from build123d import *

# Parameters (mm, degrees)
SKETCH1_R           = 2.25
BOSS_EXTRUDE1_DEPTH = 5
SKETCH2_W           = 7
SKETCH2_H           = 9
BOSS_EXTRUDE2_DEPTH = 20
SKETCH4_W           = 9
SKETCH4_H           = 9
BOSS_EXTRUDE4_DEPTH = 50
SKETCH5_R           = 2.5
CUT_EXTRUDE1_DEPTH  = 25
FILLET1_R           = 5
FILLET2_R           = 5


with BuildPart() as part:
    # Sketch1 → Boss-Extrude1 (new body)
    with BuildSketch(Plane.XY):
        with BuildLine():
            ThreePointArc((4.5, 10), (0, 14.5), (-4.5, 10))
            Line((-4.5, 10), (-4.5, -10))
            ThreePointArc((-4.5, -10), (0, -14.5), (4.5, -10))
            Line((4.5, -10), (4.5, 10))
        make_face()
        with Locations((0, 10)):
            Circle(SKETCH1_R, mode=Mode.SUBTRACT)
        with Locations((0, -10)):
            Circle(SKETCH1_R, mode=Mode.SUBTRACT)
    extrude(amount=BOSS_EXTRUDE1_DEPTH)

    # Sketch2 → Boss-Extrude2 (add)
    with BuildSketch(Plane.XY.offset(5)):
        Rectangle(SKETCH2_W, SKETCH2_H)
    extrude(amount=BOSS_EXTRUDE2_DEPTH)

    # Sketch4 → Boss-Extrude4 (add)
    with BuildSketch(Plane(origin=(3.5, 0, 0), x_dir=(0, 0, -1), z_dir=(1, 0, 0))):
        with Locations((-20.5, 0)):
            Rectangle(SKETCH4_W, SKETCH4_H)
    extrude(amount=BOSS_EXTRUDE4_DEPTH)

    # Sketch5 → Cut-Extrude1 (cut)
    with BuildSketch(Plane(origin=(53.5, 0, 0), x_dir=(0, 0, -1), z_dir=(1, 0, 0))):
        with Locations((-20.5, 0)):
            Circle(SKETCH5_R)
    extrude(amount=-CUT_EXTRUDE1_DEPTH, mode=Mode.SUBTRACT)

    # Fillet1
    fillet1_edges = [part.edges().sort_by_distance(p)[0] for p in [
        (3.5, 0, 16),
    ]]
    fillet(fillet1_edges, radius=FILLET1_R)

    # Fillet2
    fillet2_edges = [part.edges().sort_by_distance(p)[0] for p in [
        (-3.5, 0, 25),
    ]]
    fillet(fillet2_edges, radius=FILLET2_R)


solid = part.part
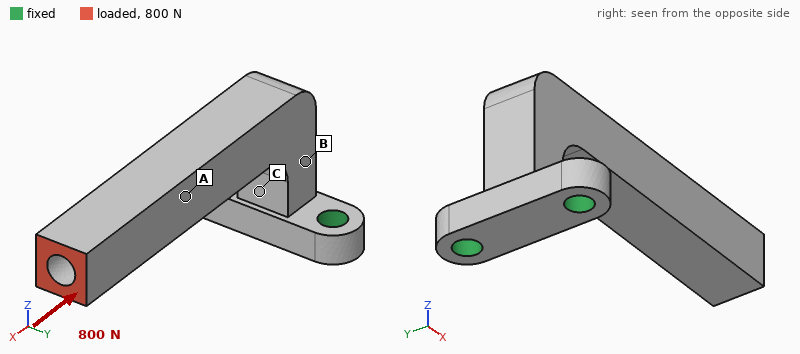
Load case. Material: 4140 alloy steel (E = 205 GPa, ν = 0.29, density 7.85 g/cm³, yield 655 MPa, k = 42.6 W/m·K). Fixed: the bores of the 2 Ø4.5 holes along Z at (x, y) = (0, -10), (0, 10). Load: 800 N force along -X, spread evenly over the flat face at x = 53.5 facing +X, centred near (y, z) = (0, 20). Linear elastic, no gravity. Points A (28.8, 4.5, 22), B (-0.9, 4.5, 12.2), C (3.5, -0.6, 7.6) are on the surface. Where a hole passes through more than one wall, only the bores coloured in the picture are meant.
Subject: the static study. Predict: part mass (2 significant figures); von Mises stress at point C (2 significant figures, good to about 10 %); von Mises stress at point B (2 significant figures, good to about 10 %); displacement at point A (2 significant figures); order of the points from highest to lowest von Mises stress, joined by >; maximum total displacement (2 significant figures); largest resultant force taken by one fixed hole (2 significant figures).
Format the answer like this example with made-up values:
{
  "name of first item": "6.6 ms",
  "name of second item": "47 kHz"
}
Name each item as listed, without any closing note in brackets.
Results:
{
  "part mass": "46 g",
  "von Mises stress at point C": "130 MPa",
  "von Mises stress at point B": "50 MPa",
  "displacement at point A": "0.12 mm",
  "order of the points from highest to lowest von Mises stress, joined by >": "C > B > A",
  "maximum total displacement": "0.21 mm",
  "largest resultant force taken by one fixed hole": "400 N"
}
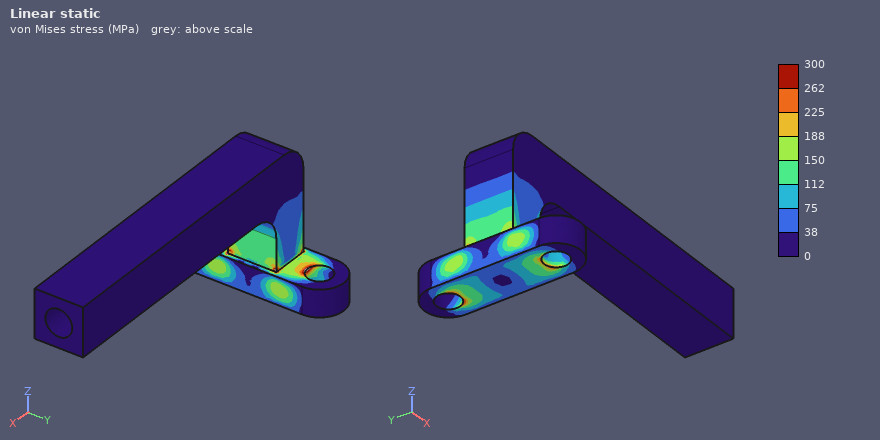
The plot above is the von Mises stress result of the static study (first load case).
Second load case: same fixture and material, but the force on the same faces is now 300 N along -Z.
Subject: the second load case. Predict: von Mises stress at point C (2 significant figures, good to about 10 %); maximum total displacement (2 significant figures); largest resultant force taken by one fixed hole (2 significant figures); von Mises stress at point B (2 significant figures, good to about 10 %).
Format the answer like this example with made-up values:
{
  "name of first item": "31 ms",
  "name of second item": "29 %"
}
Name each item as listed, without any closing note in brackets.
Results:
{
  "von Mises stress at point C": "200 MPa",
  "maximum total displacement": "0.44 mm",
  "largest resultant force taken by one fixed hole": "150 N",
  "von Mises stress at point B": "68 MPa"
}
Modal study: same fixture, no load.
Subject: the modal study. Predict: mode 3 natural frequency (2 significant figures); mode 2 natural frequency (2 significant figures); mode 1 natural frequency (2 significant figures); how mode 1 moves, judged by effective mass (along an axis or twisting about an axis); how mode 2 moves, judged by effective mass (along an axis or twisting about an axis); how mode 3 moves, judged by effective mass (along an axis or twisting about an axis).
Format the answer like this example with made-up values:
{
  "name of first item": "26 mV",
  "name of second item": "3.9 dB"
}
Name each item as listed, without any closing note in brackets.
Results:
{
  "mode 3 natural frequency": "5800 Hz",
  "mode 2 natural frequency": "1600 Hz",
  "mode 1 natural frequency": "1400 Hz",
  "how mode 1 moves, judged by effective mass": "along Z",
  "how mode 2 moves, judged by effective mass": "along Y",
  "how mode 3 moves, judged by effective mass": "along X"
}
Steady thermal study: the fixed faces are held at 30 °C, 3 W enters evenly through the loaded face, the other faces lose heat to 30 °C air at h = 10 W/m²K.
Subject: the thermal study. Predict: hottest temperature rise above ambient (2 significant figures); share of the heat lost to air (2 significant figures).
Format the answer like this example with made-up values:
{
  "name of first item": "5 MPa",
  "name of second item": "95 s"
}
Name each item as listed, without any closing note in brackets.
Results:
{
  "hottest temperature rise above ambient": "57 K",
  "share of the heat lost to air": "28 %"
}
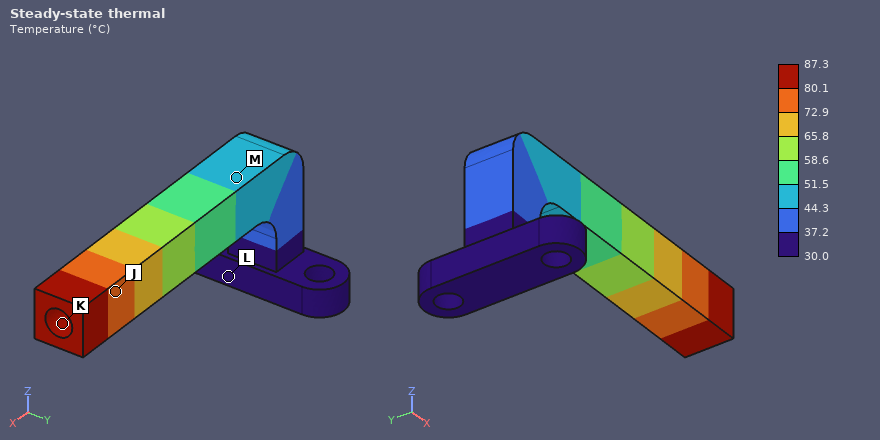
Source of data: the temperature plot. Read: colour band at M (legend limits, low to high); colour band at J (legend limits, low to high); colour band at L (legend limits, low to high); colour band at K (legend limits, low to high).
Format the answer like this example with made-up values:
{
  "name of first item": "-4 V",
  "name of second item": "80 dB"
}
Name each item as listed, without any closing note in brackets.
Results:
{
  "colour band at M": "44.3 to 51.5 °C",
  "colour band at J": "72.9 to 80.1 °C",
  "colour band at L": "30.0 to 37.2 °C",
  "colour band at K": "80.1 to 87.3 °C"
}
